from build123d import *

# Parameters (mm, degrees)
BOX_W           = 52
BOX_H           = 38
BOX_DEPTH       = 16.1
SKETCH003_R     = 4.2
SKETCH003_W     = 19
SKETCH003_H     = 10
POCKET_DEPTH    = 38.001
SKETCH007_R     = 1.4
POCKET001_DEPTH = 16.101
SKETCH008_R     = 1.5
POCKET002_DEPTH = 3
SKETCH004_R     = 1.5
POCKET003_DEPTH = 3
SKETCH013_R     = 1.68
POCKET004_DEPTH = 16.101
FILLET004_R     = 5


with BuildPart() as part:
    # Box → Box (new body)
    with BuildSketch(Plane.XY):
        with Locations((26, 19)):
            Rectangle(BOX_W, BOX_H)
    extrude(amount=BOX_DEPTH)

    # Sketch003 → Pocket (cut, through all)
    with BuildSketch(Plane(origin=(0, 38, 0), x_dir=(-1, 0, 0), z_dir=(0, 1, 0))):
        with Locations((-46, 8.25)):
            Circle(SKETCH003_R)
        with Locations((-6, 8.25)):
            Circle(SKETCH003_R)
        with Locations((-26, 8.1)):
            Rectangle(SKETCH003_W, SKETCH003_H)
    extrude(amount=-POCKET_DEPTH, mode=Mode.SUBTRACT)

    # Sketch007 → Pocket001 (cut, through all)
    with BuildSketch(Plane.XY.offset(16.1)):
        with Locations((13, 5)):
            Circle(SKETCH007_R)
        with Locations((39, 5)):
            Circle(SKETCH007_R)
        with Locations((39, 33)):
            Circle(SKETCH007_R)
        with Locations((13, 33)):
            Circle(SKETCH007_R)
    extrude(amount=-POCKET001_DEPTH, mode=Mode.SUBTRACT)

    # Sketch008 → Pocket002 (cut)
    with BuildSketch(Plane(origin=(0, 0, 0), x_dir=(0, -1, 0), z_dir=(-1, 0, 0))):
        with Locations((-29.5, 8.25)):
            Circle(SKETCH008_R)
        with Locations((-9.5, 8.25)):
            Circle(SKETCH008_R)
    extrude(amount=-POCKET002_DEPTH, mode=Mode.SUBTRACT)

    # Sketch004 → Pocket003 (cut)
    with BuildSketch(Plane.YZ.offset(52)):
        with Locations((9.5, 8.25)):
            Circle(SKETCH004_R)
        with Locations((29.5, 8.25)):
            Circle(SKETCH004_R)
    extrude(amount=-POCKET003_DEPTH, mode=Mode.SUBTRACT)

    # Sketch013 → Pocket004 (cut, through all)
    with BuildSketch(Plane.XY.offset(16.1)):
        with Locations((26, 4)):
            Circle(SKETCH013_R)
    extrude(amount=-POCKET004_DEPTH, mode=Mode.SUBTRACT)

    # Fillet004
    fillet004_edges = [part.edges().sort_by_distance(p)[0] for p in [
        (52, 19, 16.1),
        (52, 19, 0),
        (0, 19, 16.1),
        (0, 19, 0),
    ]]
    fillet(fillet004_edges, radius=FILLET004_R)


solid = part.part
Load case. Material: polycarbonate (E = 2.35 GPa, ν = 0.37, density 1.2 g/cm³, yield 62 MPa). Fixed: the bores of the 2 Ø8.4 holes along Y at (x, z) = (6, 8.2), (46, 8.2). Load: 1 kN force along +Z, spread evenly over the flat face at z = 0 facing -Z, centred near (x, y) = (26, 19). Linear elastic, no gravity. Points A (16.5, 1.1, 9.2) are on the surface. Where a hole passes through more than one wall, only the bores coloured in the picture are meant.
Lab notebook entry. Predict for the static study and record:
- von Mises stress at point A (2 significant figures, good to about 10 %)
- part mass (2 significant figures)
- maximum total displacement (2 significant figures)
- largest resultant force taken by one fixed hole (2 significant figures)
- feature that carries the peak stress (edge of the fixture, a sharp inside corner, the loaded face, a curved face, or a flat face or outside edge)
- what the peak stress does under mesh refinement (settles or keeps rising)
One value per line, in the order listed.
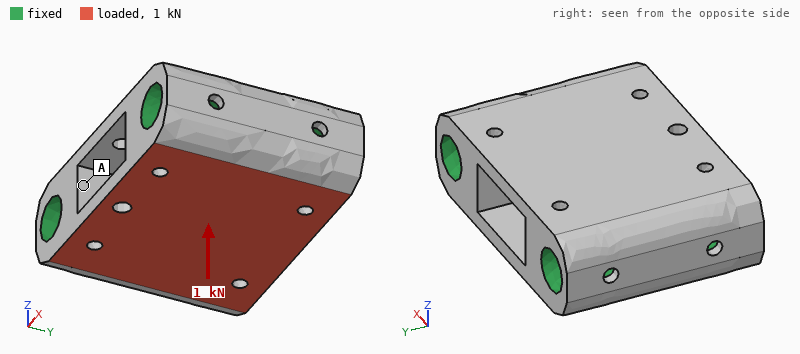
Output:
0.92 MPa
23 g
0.10 mm
520 N
a sharp inside corner
keeps rising
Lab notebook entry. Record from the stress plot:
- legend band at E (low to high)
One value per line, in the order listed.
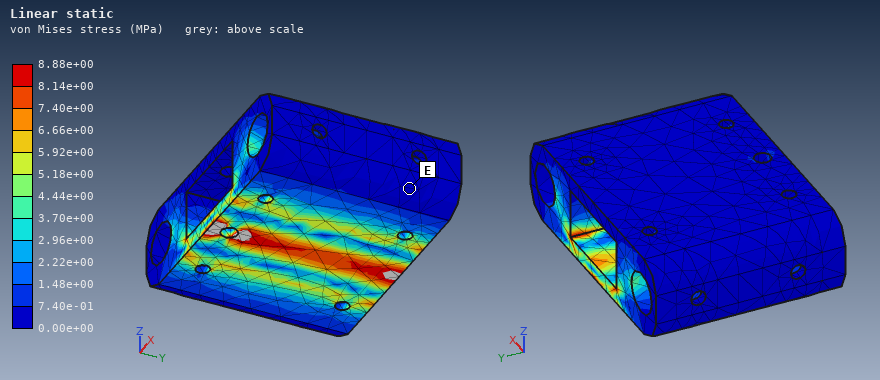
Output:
0.00e+00 to 7.40e-01 MPa
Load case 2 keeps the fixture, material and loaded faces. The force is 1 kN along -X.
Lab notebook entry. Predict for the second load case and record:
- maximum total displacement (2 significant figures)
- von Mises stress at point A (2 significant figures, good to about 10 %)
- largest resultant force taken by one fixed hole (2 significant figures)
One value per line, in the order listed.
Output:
16 µm
0.75 MPa
500 N
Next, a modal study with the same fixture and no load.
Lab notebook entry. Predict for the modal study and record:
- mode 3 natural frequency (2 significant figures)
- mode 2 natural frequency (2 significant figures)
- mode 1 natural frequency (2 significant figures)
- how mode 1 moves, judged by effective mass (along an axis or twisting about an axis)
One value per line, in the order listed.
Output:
8200 Hz
8000 Hz
7600 Hz
along Z
